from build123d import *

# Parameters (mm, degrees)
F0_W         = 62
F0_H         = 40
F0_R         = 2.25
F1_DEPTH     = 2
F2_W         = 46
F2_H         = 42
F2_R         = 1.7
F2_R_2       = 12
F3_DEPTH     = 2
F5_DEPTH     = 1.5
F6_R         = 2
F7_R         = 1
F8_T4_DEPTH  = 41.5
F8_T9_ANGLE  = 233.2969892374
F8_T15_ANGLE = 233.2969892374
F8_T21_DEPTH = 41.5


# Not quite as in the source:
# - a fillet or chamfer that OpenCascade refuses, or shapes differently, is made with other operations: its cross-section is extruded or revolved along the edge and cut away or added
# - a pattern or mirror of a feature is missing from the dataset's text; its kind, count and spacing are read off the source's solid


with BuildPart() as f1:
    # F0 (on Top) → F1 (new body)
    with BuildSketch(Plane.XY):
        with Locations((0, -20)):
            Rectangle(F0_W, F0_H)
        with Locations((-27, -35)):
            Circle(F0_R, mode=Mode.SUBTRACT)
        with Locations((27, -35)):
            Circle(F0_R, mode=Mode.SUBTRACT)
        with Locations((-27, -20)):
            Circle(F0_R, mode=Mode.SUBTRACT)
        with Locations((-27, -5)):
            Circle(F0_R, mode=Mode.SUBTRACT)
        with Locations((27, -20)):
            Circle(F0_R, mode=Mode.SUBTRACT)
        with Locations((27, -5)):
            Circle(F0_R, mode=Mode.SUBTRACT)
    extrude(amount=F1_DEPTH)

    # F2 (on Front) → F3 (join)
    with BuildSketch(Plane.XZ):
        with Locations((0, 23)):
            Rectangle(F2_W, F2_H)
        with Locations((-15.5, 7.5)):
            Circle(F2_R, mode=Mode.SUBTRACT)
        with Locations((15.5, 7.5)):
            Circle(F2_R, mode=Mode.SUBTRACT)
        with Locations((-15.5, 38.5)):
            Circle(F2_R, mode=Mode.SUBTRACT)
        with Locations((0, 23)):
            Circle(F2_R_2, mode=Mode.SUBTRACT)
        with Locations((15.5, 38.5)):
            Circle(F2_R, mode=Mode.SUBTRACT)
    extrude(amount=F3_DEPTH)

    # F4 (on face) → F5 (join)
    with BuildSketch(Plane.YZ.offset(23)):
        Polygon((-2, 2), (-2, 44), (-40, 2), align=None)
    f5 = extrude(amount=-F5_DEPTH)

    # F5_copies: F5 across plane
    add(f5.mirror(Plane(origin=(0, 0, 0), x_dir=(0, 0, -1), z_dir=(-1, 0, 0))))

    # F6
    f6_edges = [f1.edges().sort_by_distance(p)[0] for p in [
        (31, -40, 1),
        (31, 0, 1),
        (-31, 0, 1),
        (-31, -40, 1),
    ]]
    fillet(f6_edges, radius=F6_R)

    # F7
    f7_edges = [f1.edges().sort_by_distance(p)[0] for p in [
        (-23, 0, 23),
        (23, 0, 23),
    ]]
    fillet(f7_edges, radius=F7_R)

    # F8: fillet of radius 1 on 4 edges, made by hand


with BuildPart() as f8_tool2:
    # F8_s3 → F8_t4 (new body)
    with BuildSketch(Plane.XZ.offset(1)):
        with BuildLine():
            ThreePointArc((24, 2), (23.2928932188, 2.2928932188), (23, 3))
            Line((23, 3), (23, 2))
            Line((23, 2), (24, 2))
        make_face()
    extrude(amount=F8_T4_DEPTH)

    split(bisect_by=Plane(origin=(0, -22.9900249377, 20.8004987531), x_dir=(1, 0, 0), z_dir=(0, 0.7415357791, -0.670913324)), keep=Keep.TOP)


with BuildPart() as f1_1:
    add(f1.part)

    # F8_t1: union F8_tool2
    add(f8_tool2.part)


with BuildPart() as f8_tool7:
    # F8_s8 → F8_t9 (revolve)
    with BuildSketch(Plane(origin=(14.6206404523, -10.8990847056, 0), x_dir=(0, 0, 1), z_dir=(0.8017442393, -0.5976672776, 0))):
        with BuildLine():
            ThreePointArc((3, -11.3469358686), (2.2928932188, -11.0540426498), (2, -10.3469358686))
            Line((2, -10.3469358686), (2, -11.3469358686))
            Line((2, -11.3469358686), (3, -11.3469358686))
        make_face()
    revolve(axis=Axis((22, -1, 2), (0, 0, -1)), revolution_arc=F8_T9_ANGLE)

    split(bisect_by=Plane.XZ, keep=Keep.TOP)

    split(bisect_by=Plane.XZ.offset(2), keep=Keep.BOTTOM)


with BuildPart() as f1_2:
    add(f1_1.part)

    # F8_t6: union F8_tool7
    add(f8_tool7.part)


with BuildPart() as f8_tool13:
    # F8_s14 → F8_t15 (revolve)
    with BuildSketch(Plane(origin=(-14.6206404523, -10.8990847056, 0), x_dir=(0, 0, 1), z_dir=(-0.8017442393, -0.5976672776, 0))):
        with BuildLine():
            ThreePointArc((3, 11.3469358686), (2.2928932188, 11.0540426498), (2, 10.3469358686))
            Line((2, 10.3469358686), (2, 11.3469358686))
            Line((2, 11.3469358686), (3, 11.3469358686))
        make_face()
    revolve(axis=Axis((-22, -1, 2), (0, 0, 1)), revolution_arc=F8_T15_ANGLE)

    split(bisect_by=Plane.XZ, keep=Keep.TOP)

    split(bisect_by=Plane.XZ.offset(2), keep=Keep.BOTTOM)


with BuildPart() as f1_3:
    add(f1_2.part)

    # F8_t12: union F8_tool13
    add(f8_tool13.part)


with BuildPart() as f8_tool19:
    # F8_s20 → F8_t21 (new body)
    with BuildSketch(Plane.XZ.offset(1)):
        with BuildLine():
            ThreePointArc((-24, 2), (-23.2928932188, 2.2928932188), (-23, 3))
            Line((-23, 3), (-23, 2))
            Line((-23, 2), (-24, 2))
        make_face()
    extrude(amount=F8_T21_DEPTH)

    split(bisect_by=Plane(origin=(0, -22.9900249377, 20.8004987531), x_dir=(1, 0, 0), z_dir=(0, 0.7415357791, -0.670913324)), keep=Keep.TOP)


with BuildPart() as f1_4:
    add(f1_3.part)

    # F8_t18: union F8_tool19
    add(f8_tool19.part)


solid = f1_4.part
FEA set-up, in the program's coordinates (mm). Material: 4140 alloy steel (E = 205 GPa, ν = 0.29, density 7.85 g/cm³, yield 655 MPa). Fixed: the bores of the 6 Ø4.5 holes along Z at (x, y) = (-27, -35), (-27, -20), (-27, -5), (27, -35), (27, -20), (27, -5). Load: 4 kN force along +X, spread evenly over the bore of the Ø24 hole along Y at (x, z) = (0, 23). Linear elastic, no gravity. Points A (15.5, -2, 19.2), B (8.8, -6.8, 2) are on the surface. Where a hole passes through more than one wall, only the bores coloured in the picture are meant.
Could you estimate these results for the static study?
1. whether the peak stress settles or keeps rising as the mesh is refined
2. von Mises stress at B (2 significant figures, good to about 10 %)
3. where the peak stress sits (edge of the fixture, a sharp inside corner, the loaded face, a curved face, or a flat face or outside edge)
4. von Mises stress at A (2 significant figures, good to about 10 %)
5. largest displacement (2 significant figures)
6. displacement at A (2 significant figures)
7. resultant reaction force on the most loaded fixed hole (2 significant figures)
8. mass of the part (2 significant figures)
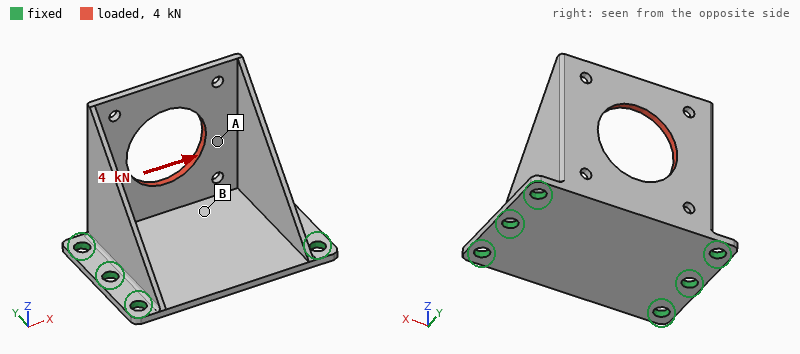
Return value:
keeps rising
39 MPa
edge of the fixture
110 MPa
83 µm
35 µm
2.4 kN
79 g
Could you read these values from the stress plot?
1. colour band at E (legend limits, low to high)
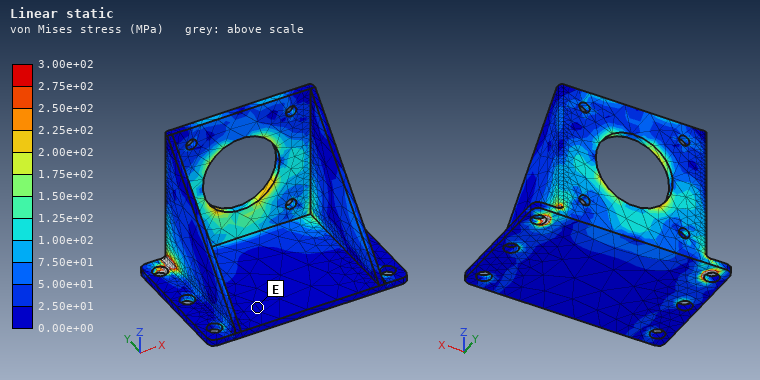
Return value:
0.00e+00 to 2.50e+01 MPa
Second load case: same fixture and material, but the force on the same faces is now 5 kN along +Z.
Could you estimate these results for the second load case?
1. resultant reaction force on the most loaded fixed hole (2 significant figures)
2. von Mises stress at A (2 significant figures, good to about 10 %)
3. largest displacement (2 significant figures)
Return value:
2.8 kN
80 MPa
74 µm
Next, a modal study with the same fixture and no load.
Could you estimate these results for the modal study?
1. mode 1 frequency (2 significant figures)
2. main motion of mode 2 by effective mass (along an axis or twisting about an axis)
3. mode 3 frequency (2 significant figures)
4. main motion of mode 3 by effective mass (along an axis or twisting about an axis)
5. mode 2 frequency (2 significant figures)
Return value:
3000 Hz
along Z
5100 Hz
along X
4500 Hz
